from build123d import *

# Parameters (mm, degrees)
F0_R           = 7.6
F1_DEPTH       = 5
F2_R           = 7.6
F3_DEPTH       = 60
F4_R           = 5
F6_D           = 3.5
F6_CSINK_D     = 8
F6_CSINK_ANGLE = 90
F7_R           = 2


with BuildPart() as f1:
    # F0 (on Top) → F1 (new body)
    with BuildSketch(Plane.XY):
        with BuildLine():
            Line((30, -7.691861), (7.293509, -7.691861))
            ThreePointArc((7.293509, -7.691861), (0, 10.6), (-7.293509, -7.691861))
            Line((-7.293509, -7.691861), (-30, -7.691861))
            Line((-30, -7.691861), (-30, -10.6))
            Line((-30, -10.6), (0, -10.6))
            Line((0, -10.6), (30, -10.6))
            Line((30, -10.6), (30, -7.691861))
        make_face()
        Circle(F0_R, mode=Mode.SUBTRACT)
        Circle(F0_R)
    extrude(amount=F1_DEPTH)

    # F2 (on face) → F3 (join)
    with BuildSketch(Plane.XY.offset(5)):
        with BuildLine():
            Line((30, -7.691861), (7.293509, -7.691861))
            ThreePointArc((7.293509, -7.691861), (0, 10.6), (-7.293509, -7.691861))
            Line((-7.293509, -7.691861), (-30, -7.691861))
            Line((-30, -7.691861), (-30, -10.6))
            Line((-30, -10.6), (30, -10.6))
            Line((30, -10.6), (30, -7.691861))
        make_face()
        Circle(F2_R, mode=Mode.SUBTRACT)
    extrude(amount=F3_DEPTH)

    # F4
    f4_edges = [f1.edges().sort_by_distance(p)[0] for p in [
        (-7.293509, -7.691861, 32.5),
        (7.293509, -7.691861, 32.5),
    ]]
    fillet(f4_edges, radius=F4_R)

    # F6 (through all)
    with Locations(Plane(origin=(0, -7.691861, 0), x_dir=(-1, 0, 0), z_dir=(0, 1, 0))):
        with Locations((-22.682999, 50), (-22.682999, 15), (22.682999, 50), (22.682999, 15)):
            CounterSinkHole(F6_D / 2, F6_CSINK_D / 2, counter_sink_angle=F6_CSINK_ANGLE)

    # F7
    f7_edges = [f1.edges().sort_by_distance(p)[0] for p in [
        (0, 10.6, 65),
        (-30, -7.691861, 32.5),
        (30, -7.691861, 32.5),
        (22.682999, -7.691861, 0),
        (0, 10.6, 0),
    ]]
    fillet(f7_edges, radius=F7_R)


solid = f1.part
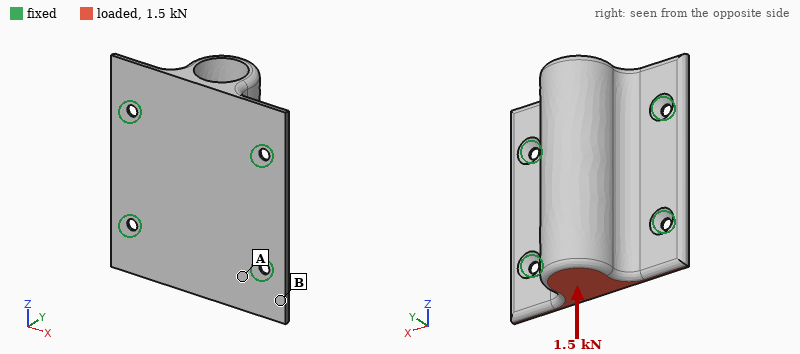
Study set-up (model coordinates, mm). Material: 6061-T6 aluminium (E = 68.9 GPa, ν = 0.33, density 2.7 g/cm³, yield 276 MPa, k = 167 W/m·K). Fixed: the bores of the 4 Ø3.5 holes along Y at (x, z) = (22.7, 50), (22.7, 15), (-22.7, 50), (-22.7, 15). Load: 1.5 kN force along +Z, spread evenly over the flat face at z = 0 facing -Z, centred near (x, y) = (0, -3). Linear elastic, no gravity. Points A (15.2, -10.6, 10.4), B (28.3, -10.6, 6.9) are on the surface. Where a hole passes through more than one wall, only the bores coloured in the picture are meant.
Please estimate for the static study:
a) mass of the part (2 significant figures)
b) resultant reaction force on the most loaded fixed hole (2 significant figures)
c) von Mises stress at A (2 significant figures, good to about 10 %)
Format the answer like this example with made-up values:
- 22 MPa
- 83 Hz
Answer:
- 61 g
- 470 N
- 16 MPa
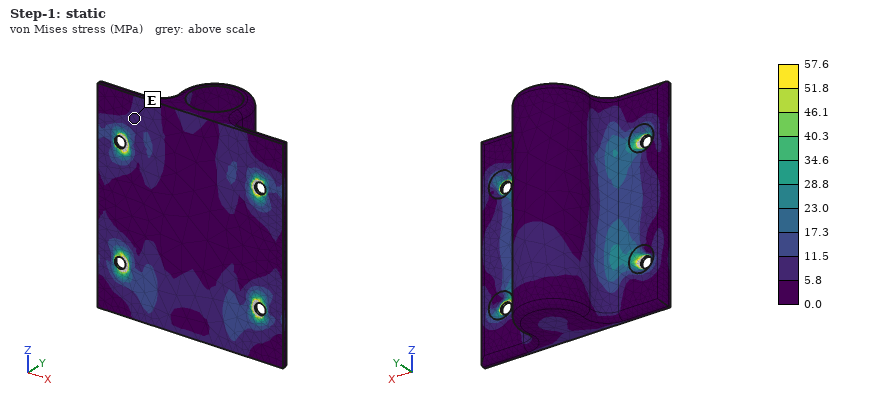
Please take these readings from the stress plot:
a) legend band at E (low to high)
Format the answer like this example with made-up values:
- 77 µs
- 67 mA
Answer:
- 5.8 to 11.5 MPa
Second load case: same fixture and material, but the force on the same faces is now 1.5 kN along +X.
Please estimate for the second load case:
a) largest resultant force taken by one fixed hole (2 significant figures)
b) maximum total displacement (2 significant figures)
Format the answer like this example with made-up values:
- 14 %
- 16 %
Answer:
- 800 N
- 17 µm
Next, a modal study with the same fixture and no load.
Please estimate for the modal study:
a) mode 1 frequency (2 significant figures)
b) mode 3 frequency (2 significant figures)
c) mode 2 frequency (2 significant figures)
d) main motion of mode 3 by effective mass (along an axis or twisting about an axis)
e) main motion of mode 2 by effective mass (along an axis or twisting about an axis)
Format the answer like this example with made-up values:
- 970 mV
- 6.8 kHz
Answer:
- 4000 Hz
- 7900 Hz
- 4800 Hz
- along X
- along Y
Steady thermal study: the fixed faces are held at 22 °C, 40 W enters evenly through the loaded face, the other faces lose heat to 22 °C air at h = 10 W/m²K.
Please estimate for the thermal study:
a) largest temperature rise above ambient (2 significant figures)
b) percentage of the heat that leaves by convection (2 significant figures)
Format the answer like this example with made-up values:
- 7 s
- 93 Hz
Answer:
- 33 K
- 4.3 %
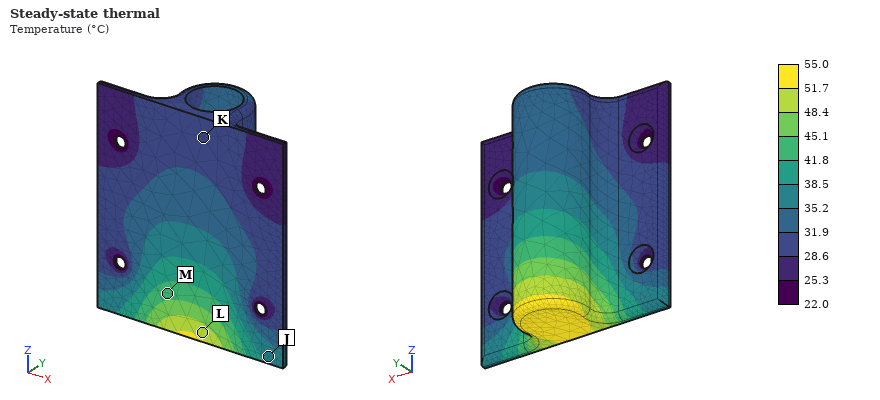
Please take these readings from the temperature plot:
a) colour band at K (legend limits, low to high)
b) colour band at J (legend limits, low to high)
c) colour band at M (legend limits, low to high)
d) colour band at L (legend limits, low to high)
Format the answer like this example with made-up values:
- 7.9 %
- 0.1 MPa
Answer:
- 28.6 to 31.9 °C
- 35.2 to 38.5 °C
- 41.8 to 45.1 °C
- 48.4 to 51.7 °C
